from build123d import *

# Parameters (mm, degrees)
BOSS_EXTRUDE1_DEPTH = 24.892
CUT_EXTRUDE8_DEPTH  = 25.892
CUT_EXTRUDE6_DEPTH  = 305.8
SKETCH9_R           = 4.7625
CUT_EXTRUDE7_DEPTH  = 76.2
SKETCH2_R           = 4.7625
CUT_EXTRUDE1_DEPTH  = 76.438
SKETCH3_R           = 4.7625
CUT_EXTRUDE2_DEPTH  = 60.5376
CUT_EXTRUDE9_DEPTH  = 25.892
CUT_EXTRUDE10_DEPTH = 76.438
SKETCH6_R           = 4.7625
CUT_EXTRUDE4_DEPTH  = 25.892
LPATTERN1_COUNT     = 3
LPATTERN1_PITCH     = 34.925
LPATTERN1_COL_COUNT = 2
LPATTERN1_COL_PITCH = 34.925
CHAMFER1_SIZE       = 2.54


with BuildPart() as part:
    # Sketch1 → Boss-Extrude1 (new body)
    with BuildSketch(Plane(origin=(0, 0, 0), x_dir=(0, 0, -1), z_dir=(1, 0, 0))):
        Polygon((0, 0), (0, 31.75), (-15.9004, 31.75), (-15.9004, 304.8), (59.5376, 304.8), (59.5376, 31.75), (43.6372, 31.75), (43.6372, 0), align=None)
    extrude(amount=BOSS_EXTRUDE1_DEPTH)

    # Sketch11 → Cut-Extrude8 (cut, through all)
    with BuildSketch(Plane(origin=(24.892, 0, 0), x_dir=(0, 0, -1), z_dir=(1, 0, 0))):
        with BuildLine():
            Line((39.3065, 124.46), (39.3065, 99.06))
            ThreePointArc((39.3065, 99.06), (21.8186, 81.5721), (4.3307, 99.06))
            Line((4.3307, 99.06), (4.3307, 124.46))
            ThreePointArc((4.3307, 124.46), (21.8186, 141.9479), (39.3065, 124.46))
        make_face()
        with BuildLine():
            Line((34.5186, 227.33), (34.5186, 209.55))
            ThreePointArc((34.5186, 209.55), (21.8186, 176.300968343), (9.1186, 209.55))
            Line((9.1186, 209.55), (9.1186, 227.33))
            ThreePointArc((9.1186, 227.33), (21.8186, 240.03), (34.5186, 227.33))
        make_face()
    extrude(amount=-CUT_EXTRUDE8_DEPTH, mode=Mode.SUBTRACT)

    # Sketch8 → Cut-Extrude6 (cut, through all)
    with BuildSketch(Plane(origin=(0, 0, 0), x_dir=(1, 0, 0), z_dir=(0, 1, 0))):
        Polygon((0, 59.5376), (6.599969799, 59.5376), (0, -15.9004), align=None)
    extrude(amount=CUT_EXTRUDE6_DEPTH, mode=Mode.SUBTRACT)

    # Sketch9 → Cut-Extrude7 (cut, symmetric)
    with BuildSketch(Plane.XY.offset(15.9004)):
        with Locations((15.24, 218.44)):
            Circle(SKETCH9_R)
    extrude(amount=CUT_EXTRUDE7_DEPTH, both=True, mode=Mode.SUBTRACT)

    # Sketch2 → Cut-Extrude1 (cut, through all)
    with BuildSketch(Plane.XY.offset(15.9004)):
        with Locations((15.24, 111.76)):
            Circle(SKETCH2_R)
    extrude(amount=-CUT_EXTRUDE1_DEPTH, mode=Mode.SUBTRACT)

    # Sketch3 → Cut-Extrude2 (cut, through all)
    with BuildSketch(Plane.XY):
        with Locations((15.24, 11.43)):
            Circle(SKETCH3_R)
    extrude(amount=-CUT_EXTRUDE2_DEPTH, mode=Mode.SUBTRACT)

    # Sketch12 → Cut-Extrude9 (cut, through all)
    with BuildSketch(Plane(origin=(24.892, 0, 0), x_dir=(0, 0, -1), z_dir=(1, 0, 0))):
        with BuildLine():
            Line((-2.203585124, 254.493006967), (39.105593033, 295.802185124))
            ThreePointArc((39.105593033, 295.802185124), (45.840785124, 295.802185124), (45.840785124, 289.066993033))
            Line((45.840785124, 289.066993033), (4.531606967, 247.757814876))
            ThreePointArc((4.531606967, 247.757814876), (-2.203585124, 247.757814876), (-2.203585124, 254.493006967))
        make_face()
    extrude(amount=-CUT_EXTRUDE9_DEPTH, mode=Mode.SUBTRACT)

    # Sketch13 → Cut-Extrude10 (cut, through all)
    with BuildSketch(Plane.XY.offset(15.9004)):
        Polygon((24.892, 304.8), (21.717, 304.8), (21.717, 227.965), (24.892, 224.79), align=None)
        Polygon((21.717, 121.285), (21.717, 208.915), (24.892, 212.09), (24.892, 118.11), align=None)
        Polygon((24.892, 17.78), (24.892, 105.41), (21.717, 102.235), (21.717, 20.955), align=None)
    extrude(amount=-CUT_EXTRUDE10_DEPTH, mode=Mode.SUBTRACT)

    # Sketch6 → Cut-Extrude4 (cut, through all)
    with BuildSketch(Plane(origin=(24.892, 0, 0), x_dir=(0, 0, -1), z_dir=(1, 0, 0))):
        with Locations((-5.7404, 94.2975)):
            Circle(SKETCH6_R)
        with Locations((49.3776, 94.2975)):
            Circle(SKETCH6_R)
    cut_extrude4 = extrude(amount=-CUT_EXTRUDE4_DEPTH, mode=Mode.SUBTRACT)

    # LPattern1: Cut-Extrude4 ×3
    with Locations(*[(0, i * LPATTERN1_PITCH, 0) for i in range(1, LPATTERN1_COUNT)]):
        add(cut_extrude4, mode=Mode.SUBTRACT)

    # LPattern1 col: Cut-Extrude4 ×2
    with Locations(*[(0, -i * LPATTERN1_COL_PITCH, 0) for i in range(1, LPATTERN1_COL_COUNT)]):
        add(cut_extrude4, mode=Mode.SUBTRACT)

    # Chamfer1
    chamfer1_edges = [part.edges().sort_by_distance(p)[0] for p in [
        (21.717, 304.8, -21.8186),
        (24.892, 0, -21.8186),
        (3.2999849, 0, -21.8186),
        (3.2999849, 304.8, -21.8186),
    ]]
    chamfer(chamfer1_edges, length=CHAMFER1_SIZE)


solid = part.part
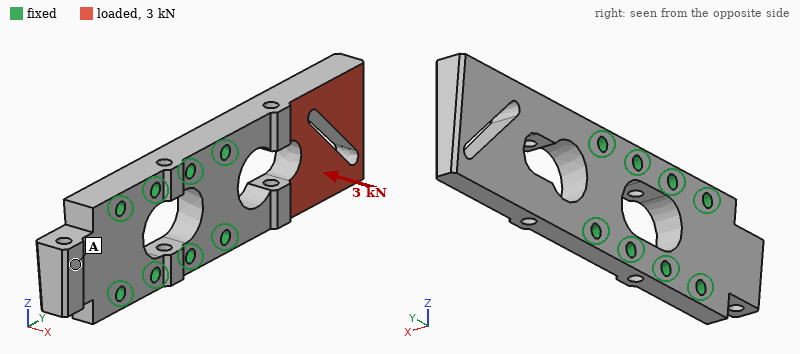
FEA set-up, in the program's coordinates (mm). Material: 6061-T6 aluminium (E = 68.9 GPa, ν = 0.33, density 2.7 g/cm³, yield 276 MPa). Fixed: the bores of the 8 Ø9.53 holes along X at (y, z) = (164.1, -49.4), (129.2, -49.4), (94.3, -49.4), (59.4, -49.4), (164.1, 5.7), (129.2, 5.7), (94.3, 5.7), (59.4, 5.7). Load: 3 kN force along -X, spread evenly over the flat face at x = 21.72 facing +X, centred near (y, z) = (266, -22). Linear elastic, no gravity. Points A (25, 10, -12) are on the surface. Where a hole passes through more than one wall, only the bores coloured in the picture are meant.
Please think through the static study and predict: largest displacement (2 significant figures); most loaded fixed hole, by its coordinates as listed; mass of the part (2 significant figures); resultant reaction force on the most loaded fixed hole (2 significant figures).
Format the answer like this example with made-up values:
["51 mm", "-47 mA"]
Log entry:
["1.0 mm", "(164.1, 5.7)", "850 g", "2.7 kN"]
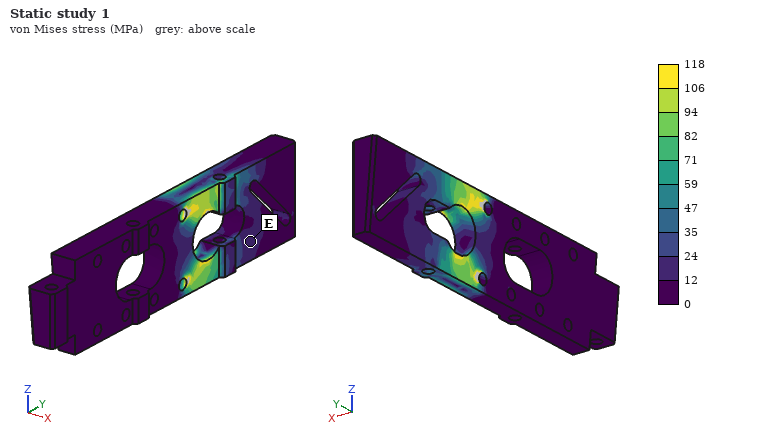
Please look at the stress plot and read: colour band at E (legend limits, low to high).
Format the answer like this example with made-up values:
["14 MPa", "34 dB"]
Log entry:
["12 to 24 MPa"]
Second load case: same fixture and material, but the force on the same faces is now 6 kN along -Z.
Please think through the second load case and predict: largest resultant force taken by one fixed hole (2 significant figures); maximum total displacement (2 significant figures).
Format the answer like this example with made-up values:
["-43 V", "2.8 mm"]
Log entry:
["9.9 kN", "0.32 mm"]
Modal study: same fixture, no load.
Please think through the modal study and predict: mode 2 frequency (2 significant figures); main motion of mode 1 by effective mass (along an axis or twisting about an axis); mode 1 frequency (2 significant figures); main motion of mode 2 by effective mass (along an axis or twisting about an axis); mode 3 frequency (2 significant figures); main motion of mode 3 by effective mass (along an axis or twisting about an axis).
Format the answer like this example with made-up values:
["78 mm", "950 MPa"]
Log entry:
["1800 Hz", "along X", "660 Hz", "along Z", "2000 Hz", "twisting about Y"]
